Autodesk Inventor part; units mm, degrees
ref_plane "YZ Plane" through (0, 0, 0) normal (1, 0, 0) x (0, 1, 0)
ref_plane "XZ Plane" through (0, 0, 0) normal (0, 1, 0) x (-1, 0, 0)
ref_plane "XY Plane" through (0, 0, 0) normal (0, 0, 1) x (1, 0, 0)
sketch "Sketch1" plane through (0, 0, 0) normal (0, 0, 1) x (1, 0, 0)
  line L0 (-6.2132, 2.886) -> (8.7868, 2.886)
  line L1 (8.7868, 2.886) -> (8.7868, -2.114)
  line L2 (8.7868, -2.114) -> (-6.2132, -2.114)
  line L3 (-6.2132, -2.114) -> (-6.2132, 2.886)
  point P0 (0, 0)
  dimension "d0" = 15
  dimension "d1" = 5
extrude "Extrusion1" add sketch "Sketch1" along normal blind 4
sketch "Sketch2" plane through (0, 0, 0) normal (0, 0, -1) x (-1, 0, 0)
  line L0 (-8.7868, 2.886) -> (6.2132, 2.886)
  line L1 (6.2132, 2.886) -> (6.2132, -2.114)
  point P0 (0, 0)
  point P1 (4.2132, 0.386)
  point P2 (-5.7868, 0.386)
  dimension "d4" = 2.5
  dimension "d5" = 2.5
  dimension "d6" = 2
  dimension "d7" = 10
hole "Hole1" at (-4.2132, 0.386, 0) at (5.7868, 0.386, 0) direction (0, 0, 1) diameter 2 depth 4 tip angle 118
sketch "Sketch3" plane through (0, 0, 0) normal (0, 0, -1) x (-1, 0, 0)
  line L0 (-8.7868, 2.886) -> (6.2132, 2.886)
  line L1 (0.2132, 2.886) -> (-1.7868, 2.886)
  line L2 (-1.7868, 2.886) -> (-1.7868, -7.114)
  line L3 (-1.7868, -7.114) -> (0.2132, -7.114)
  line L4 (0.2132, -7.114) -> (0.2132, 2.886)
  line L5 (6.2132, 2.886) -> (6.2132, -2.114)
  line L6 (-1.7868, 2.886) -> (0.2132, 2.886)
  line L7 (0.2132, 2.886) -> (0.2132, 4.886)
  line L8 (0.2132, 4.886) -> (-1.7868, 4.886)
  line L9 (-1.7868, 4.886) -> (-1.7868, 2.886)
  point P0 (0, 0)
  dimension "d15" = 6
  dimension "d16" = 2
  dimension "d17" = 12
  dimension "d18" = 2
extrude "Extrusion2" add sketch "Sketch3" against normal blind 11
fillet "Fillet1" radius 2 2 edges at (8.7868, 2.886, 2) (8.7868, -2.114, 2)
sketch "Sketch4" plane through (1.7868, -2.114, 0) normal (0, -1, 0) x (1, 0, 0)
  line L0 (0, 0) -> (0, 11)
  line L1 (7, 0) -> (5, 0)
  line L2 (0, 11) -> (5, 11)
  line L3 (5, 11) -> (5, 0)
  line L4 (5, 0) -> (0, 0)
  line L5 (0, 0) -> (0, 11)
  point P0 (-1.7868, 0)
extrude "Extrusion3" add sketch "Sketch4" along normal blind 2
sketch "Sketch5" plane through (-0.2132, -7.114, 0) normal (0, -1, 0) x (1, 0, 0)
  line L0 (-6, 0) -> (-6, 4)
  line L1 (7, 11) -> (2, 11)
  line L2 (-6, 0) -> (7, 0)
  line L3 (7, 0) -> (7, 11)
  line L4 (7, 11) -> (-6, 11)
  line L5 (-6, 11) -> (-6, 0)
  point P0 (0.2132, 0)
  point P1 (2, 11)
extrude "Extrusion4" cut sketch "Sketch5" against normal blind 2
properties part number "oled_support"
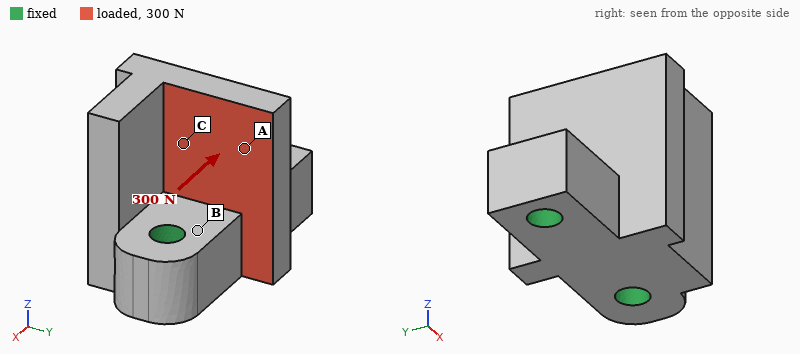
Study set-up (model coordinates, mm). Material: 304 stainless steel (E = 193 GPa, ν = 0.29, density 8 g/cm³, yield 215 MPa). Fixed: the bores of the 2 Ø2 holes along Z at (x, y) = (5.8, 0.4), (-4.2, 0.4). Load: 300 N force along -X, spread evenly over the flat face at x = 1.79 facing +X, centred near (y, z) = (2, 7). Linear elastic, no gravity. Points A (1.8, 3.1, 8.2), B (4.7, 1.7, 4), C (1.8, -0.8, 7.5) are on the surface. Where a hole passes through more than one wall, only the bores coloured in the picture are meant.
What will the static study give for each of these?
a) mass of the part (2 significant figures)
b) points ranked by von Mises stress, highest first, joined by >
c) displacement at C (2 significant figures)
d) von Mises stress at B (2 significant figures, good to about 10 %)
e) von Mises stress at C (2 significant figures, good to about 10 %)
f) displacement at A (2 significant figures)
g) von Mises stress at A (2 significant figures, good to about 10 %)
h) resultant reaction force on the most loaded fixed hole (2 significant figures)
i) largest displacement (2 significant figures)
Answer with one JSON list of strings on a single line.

["4.5 g", "C > A > B", "3.0 µm", "11 MPa", "51 MPa", "6.9 µm", "29 MPa", "220 N", "13 µm"]
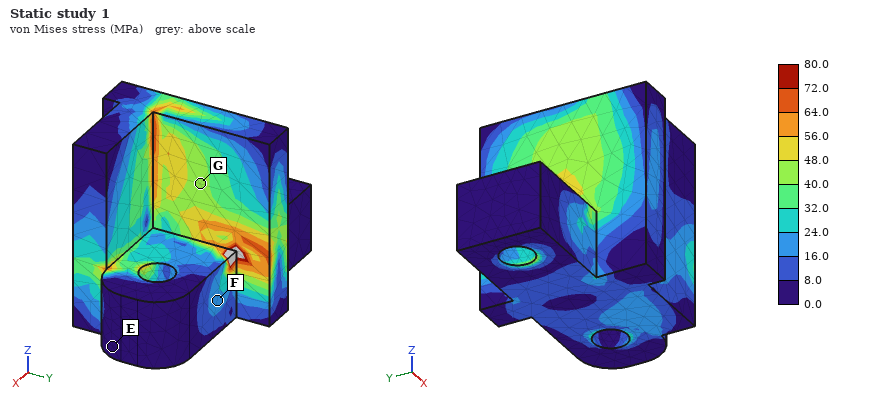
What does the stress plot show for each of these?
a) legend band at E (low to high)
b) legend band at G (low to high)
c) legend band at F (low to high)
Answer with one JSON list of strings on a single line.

["0.0 to 8.0 MPa", "40.0 to 48.0 MPa", "16.0 to 24.0 MPa"]
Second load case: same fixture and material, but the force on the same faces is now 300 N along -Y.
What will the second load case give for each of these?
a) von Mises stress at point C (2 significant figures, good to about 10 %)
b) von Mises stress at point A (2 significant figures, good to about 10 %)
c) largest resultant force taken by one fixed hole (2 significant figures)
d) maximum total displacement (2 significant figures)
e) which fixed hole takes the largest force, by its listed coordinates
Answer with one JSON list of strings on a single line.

["36 MPa", "26 MPa", "180 N", "7.9 µm", "(5.8, 0.4)"]
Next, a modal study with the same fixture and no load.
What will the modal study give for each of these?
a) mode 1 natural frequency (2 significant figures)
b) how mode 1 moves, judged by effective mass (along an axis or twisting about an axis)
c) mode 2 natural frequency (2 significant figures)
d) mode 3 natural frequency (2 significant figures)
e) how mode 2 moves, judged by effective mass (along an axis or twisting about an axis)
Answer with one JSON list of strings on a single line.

["26 kHz", "along Y", "33 kHz", "46 kHz", "along X"]
